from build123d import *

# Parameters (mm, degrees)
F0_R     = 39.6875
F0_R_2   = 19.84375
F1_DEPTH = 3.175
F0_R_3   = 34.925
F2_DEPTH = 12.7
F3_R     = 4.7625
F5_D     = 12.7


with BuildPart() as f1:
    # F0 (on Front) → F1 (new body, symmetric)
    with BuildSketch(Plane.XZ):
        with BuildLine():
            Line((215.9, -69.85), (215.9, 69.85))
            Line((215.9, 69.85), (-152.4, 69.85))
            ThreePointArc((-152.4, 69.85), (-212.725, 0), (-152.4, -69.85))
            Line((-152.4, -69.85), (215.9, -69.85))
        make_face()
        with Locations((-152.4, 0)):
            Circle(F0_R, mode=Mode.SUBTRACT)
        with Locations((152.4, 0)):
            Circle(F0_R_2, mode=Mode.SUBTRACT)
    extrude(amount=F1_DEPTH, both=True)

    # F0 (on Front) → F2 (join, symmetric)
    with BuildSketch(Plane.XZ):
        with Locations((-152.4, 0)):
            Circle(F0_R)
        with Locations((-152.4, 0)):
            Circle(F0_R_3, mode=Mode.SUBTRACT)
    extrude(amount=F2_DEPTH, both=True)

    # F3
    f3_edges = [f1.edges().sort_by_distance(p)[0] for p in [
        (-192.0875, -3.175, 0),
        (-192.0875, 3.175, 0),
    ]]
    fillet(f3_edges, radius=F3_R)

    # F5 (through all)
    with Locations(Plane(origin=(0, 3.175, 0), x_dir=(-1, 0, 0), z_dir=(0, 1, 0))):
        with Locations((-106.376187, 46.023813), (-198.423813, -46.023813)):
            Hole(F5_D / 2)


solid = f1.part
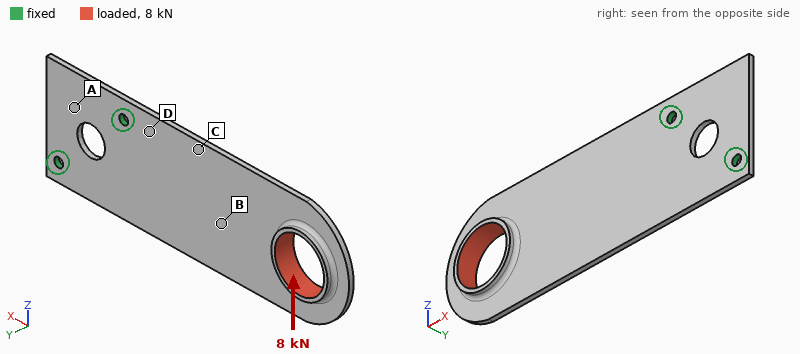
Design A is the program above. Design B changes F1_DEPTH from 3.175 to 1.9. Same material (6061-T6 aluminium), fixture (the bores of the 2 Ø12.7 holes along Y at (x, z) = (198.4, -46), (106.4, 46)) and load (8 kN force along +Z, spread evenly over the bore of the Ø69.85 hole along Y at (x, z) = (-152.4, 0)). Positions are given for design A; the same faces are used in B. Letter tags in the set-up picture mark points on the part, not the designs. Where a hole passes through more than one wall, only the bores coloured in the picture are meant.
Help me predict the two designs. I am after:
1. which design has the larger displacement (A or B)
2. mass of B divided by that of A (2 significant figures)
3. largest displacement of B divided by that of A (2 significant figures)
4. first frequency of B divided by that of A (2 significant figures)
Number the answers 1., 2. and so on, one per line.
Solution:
1. B
2. 0.63
3. 1.7
4. 0.55
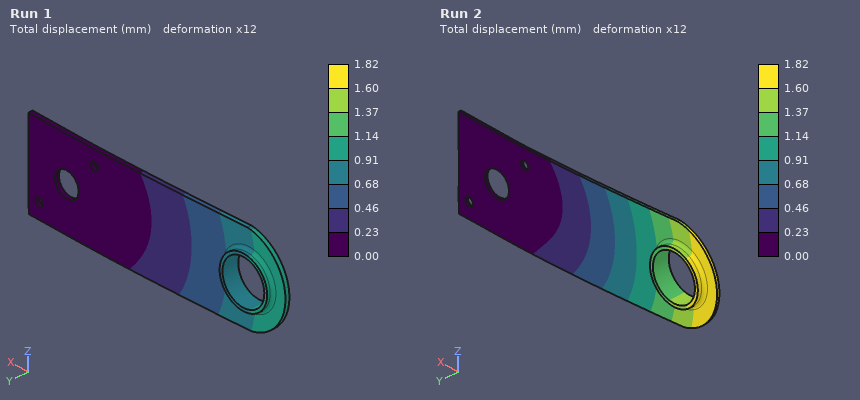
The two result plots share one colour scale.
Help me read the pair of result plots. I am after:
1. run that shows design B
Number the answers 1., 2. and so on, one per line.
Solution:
1. Run 2
